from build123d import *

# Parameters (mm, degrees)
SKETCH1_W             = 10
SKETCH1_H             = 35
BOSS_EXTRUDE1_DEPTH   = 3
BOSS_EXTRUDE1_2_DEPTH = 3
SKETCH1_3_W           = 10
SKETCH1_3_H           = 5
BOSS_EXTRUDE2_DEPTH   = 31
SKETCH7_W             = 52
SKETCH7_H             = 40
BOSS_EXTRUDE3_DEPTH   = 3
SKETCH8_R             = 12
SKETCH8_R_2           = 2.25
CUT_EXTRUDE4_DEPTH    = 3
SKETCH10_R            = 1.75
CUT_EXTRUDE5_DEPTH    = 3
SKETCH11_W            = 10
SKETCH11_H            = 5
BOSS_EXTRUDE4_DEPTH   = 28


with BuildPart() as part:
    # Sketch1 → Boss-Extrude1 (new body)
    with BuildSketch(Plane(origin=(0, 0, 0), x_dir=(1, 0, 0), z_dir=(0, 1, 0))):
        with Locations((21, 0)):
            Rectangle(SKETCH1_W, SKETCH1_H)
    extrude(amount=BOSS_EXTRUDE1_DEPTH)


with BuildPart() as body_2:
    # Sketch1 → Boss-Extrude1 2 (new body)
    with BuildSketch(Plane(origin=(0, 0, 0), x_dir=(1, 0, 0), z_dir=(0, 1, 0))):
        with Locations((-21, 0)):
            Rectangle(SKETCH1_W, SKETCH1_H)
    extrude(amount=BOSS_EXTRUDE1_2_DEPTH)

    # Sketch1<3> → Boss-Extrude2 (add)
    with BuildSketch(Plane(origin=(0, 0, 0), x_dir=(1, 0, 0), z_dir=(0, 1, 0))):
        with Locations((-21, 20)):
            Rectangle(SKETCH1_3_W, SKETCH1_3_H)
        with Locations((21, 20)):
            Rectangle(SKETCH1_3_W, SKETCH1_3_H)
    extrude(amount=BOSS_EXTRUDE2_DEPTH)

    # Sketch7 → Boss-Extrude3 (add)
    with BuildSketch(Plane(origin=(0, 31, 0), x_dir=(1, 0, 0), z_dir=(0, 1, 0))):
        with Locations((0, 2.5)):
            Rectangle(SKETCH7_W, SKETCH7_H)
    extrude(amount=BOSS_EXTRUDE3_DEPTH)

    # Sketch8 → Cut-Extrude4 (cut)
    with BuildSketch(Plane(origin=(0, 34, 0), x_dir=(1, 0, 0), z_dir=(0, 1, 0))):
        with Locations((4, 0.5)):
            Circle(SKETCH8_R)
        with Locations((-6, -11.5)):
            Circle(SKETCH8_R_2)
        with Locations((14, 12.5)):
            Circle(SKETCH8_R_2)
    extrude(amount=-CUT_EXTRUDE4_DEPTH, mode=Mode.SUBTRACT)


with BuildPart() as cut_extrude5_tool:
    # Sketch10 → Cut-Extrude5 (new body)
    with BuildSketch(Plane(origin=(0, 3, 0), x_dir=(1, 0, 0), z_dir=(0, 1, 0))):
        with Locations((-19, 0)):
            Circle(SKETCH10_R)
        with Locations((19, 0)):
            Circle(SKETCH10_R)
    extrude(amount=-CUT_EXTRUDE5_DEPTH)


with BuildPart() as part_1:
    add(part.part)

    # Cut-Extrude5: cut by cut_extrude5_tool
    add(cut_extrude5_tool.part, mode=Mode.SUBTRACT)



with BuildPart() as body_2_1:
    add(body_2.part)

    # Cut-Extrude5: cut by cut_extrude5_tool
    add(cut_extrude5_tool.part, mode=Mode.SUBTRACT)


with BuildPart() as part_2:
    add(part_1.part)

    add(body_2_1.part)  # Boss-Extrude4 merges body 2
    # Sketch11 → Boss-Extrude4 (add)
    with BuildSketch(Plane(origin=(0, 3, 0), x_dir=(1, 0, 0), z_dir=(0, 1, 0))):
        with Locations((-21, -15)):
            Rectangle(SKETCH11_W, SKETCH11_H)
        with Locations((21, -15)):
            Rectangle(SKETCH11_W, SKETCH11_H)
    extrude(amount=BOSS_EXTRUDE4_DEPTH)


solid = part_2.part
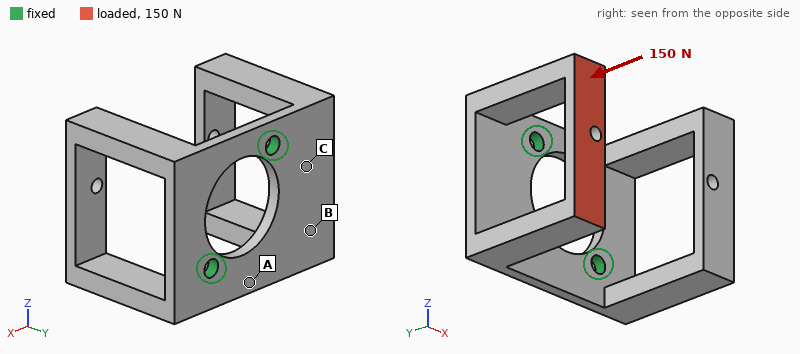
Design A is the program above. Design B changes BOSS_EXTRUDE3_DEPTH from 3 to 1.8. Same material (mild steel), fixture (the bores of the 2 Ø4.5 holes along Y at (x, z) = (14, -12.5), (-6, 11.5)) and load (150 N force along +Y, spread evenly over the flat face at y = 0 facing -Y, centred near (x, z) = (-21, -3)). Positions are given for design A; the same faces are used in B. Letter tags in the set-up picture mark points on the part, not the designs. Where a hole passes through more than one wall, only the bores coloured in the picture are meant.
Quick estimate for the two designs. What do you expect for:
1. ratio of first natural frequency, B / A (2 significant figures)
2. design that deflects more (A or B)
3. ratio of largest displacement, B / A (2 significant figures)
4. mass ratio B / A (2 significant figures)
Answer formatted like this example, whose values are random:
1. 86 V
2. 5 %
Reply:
1. 0.52
2. B
3. 4.0
4. 0.85
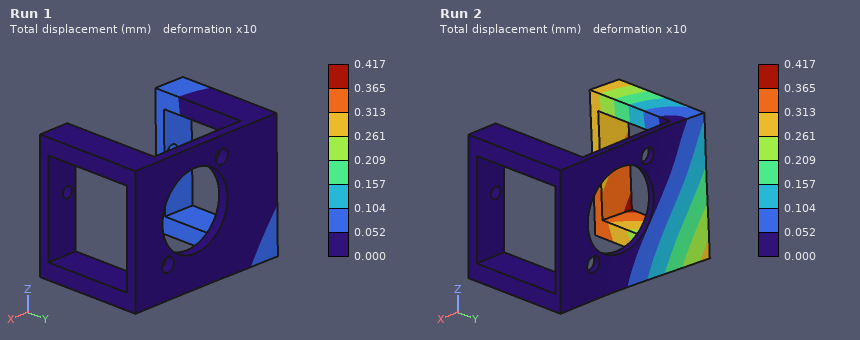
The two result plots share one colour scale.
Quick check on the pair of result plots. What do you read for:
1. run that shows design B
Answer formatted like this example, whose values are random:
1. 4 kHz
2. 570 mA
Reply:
1. Run 2
